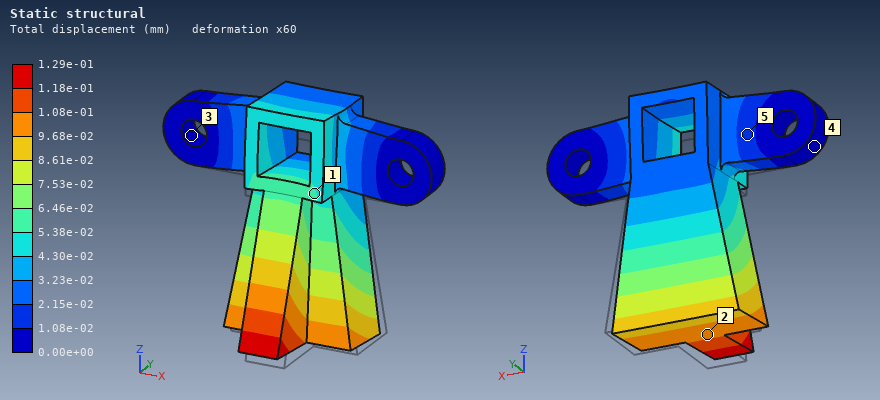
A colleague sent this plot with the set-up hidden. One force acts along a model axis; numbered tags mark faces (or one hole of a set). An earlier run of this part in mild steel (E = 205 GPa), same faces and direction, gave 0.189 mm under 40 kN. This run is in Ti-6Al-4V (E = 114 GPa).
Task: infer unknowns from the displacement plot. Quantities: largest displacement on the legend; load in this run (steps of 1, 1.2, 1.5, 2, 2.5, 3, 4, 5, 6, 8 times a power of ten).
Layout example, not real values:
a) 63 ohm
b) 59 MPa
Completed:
a) 1.29e-01 mm
b) 15 kN
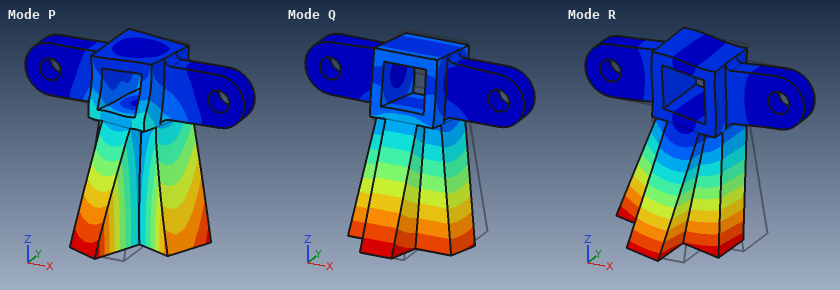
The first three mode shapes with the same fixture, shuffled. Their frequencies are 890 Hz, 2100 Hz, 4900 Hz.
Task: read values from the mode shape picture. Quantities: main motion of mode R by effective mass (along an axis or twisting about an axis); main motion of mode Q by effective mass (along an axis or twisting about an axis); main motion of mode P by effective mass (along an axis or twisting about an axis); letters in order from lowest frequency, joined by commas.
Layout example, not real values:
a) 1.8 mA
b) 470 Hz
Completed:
a) along X
b) along Y
c) twisting about Z
d) Q, R, P
